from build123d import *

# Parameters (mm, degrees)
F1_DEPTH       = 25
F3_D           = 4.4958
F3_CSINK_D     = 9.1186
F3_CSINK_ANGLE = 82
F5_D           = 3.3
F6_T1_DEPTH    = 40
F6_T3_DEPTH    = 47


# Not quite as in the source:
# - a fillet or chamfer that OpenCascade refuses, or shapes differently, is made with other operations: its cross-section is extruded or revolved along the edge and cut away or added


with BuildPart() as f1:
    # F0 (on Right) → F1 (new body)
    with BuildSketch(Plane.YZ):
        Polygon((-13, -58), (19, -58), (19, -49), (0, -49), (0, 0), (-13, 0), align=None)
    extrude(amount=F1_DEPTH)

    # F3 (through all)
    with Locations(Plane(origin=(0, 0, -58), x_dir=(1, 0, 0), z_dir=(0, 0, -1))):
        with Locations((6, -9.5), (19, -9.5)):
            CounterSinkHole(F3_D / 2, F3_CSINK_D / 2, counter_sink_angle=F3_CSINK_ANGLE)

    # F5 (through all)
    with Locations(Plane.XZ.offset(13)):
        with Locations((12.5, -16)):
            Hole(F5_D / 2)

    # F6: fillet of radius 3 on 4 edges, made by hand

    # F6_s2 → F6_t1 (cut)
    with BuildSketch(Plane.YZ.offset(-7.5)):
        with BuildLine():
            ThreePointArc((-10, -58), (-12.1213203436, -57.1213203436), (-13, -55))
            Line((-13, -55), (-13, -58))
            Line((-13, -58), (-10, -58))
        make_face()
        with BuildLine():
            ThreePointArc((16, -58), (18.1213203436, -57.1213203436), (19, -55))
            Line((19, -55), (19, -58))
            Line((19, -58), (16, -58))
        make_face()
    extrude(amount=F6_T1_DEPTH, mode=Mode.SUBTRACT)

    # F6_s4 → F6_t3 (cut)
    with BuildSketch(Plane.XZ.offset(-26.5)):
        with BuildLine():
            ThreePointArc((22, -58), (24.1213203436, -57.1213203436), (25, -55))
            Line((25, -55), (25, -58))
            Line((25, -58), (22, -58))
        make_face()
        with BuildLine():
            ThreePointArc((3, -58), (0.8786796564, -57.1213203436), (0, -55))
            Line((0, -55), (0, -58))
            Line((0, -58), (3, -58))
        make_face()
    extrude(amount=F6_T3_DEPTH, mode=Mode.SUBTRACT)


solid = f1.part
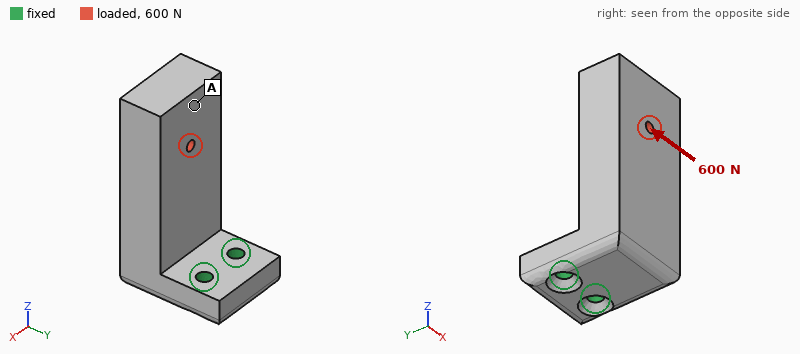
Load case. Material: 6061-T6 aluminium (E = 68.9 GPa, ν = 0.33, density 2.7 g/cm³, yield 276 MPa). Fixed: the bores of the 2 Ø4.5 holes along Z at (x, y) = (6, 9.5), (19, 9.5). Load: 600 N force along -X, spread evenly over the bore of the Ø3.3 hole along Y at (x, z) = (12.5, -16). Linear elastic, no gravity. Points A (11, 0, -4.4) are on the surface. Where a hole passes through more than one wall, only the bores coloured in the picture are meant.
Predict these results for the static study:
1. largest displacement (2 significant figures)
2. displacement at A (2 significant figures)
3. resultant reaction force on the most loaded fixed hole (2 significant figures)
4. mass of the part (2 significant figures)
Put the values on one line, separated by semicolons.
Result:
97 µm; 87 µm; 1.3 kN; 60 g
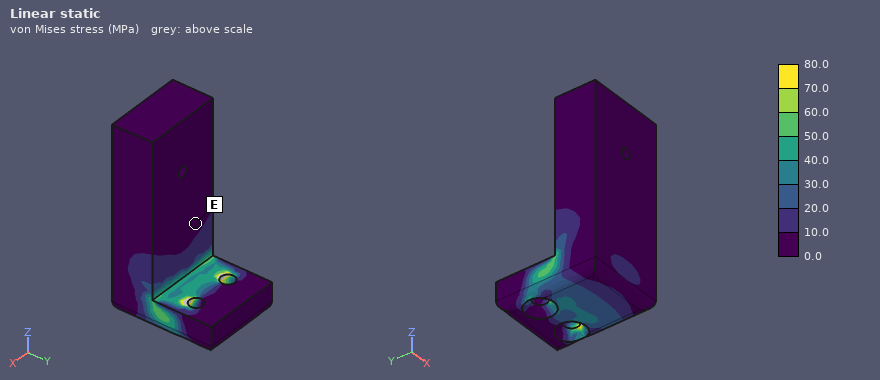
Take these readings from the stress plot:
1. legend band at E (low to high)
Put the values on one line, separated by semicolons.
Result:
0.0 to 10.0 MPa
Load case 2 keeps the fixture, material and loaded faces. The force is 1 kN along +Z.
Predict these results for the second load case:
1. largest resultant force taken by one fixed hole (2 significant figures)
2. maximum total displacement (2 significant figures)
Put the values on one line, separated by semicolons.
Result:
500 N; 92 µm
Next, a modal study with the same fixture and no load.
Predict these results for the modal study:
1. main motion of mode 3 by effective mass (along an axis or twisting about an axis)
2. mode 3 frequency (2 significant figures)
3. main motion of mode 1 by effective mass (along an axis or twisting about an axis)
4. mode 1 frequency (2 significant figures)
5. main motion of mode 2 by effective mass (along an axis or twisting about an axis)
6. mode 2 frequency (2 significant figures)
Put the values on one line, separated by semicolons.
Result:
along Z; 8100 Hz; along Y; 1700 Hz; along X; 2600 Hz
